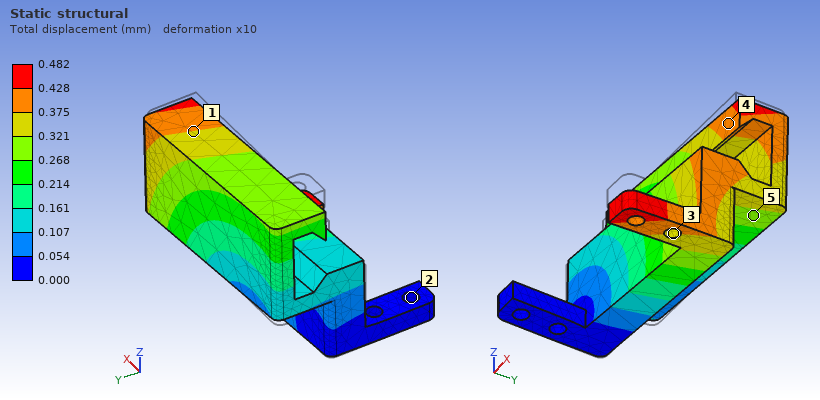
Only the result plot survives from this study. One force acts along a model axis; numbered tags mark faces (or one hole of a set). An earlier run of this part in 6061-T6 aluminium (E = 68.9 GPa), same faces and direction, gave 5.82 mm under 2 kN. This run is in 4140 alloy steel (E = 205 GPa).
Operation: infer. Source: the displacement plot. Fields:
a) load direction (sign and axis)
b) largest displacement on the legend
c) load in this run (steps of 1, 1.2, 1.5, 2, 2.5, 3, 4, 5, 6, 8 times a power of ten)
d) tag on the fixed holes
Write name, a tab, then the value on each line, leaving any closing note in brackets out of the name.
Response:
load direction	-Z
largest displacement on the legend	0.482 mm
load in this run	500 N
tag on the fixed holes	2
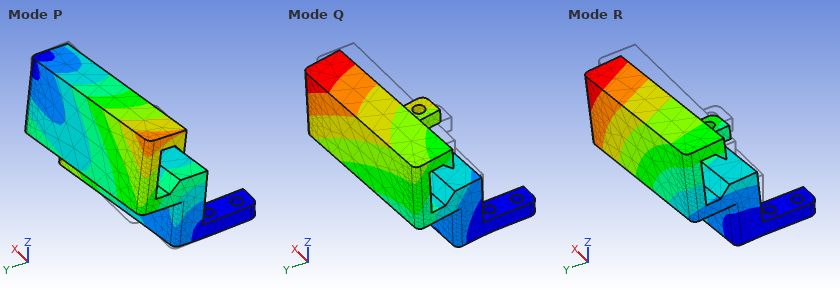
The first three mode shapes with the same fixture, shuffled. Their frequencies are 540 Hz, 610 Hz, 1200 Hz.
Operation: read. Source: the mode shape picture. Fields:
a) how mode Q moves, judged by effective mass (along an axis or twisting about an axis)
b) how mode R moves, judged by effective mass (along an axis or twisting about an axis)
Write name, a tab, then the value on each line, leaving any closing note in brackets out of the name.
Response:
how mode Q moves, judged by effective mass	along Y
how mode R moves, judged by effective mass	along Z
